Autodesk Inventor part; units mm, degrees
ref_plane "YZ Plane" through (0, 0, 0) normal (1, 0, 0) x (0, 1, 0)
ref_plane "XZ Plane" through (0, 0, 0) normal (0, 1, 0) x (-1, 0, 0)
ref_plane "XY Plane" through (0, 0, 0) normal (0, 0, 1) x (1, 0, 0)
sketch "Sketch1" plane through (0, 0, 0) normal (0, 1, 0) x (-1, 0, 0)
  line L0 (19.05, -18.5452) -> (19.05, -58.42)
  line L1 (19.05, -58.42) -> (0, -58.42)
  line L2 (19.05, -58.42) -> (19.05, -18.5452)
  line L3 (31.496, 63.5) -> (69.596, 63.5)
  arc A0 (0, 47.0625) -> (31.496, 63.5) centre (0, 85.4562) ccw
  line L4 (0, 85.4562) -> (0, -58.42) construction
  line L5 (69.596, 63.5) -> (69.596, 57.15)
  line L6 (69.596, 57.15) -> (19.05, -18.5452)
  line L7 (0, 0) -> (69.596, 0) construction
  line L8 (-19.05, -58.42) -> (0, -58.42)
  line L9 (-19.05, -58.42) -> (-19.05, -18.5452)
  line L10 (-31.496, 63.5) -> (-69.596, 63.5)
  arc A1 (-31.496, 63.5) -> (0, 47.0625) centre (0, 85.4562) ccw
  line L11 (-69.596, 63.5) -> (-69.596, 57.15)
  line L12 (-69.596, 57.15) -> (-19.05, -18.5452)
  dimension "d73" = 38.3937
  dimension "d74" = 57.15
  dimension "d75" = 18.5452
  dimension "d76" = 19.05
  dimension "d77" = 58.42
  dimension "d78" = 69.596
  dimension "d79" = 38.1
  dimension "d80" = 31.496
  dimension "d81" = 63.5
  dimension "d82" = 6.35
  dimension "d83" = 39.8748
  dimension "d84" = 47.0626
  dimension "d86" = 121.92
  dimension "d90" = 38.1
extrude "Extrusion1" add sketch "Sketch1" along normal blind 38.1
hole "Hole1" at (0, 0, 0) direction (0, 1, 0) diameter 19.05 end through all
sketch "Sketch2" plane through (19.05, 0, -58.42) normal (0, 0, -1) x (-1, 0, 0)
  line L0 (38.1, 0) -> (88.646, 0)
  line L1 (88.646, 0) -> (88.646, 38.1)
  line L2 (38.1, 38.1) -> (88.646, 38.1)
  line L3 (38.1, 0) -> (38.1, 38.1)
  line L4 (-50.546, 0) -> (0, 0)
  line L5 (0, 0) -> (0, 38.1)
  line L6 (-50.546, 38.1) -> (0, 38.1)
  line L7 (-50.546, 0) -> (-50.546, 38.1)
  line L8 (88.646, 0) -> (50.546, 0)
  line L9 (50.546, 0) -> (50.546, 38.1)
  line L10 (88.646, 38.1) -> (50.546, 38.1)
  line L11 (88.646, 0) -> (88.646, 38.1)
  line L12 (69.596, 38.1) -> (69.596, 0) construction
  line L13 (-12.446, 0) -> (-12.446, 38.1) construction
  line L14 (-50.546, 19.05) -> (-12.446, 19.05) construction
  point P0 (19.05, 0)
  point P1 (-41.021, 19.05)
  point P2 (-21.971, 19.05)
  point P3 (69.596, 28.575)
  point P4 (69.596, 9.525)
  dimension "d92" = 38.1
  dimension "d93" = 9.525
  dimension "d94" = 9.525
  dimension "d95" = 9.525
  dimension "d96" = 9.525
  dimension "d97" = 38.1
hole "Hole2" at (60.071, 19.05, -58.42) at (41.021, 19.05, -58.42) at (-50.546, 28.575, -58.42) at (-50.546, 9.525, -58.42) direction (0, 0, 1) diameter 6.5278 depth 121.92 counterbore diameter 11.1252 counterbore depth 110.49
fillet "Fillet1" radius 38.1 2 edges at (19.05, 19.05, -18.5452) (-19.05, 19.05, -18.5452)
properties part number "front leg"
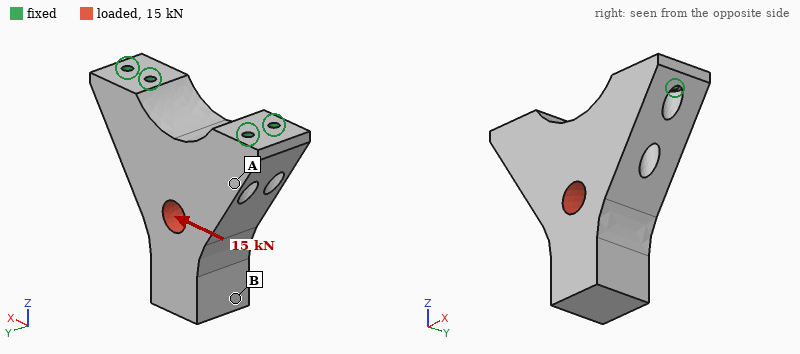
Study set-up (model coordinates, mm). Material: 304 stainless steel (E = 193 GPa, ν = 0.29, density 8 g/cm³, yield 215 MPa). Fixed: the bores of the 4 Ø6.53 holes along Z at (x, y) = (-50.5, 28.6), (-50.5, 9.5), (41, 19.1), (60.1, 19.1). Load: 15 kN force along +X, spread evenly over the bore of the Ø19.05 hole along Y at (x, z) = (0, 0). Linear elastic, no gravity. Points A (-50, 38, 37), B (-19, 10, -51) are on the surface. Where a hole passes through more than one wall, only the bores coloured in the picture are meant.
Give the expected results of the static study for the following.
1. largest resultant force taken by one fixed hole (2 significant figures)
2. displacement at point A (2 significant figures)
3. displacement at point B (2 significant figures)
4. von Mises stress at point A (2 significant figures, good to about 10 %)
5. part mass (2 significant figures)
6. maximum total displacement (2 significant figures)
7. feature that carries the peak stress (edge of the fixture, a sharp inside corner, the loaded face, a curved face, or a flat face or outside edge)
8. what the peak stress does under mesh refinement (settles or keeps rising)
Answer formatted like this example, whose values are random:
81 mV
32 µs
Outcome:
5.9 kN
2.9 µm
9.5 µm
12 MPa
2.4 kg
9.7 µm
edge of the fixture
keeps rising
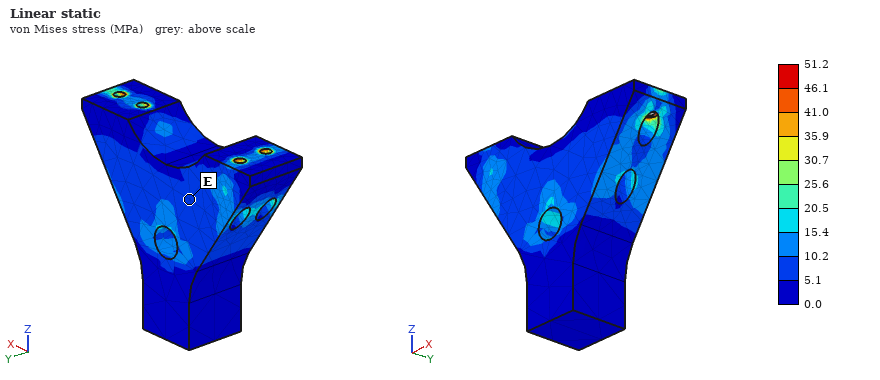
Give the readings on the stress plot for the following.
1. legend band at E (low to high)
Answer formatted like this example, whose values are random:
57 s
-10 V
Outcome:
5.1 to 10.2 MPa
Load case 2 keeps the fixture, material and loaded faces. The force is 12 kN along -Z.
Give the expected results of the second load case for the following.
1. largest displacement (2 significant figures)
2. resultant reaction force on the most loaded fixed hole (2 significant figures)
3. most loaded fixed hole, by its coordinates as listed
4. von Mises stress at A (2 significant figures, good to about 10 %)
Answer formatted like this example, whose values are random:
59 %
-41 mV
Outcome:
3.8 µm
5.0 kN
(41, 19.1)
7.1 MPa
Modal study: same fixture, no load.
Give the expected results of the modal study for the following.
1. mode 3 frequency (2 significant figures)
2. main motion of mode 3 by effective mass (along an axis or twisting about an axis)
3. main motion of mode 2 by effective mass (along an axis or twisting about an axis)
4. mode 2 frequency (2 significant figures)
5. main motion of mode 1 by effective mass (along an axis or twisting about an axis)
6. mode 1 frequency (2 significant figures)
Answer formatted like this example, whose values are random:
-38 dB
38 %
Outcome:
7100 Hz
along Y
along X
4900 Hz
along Y
1400 Hz
